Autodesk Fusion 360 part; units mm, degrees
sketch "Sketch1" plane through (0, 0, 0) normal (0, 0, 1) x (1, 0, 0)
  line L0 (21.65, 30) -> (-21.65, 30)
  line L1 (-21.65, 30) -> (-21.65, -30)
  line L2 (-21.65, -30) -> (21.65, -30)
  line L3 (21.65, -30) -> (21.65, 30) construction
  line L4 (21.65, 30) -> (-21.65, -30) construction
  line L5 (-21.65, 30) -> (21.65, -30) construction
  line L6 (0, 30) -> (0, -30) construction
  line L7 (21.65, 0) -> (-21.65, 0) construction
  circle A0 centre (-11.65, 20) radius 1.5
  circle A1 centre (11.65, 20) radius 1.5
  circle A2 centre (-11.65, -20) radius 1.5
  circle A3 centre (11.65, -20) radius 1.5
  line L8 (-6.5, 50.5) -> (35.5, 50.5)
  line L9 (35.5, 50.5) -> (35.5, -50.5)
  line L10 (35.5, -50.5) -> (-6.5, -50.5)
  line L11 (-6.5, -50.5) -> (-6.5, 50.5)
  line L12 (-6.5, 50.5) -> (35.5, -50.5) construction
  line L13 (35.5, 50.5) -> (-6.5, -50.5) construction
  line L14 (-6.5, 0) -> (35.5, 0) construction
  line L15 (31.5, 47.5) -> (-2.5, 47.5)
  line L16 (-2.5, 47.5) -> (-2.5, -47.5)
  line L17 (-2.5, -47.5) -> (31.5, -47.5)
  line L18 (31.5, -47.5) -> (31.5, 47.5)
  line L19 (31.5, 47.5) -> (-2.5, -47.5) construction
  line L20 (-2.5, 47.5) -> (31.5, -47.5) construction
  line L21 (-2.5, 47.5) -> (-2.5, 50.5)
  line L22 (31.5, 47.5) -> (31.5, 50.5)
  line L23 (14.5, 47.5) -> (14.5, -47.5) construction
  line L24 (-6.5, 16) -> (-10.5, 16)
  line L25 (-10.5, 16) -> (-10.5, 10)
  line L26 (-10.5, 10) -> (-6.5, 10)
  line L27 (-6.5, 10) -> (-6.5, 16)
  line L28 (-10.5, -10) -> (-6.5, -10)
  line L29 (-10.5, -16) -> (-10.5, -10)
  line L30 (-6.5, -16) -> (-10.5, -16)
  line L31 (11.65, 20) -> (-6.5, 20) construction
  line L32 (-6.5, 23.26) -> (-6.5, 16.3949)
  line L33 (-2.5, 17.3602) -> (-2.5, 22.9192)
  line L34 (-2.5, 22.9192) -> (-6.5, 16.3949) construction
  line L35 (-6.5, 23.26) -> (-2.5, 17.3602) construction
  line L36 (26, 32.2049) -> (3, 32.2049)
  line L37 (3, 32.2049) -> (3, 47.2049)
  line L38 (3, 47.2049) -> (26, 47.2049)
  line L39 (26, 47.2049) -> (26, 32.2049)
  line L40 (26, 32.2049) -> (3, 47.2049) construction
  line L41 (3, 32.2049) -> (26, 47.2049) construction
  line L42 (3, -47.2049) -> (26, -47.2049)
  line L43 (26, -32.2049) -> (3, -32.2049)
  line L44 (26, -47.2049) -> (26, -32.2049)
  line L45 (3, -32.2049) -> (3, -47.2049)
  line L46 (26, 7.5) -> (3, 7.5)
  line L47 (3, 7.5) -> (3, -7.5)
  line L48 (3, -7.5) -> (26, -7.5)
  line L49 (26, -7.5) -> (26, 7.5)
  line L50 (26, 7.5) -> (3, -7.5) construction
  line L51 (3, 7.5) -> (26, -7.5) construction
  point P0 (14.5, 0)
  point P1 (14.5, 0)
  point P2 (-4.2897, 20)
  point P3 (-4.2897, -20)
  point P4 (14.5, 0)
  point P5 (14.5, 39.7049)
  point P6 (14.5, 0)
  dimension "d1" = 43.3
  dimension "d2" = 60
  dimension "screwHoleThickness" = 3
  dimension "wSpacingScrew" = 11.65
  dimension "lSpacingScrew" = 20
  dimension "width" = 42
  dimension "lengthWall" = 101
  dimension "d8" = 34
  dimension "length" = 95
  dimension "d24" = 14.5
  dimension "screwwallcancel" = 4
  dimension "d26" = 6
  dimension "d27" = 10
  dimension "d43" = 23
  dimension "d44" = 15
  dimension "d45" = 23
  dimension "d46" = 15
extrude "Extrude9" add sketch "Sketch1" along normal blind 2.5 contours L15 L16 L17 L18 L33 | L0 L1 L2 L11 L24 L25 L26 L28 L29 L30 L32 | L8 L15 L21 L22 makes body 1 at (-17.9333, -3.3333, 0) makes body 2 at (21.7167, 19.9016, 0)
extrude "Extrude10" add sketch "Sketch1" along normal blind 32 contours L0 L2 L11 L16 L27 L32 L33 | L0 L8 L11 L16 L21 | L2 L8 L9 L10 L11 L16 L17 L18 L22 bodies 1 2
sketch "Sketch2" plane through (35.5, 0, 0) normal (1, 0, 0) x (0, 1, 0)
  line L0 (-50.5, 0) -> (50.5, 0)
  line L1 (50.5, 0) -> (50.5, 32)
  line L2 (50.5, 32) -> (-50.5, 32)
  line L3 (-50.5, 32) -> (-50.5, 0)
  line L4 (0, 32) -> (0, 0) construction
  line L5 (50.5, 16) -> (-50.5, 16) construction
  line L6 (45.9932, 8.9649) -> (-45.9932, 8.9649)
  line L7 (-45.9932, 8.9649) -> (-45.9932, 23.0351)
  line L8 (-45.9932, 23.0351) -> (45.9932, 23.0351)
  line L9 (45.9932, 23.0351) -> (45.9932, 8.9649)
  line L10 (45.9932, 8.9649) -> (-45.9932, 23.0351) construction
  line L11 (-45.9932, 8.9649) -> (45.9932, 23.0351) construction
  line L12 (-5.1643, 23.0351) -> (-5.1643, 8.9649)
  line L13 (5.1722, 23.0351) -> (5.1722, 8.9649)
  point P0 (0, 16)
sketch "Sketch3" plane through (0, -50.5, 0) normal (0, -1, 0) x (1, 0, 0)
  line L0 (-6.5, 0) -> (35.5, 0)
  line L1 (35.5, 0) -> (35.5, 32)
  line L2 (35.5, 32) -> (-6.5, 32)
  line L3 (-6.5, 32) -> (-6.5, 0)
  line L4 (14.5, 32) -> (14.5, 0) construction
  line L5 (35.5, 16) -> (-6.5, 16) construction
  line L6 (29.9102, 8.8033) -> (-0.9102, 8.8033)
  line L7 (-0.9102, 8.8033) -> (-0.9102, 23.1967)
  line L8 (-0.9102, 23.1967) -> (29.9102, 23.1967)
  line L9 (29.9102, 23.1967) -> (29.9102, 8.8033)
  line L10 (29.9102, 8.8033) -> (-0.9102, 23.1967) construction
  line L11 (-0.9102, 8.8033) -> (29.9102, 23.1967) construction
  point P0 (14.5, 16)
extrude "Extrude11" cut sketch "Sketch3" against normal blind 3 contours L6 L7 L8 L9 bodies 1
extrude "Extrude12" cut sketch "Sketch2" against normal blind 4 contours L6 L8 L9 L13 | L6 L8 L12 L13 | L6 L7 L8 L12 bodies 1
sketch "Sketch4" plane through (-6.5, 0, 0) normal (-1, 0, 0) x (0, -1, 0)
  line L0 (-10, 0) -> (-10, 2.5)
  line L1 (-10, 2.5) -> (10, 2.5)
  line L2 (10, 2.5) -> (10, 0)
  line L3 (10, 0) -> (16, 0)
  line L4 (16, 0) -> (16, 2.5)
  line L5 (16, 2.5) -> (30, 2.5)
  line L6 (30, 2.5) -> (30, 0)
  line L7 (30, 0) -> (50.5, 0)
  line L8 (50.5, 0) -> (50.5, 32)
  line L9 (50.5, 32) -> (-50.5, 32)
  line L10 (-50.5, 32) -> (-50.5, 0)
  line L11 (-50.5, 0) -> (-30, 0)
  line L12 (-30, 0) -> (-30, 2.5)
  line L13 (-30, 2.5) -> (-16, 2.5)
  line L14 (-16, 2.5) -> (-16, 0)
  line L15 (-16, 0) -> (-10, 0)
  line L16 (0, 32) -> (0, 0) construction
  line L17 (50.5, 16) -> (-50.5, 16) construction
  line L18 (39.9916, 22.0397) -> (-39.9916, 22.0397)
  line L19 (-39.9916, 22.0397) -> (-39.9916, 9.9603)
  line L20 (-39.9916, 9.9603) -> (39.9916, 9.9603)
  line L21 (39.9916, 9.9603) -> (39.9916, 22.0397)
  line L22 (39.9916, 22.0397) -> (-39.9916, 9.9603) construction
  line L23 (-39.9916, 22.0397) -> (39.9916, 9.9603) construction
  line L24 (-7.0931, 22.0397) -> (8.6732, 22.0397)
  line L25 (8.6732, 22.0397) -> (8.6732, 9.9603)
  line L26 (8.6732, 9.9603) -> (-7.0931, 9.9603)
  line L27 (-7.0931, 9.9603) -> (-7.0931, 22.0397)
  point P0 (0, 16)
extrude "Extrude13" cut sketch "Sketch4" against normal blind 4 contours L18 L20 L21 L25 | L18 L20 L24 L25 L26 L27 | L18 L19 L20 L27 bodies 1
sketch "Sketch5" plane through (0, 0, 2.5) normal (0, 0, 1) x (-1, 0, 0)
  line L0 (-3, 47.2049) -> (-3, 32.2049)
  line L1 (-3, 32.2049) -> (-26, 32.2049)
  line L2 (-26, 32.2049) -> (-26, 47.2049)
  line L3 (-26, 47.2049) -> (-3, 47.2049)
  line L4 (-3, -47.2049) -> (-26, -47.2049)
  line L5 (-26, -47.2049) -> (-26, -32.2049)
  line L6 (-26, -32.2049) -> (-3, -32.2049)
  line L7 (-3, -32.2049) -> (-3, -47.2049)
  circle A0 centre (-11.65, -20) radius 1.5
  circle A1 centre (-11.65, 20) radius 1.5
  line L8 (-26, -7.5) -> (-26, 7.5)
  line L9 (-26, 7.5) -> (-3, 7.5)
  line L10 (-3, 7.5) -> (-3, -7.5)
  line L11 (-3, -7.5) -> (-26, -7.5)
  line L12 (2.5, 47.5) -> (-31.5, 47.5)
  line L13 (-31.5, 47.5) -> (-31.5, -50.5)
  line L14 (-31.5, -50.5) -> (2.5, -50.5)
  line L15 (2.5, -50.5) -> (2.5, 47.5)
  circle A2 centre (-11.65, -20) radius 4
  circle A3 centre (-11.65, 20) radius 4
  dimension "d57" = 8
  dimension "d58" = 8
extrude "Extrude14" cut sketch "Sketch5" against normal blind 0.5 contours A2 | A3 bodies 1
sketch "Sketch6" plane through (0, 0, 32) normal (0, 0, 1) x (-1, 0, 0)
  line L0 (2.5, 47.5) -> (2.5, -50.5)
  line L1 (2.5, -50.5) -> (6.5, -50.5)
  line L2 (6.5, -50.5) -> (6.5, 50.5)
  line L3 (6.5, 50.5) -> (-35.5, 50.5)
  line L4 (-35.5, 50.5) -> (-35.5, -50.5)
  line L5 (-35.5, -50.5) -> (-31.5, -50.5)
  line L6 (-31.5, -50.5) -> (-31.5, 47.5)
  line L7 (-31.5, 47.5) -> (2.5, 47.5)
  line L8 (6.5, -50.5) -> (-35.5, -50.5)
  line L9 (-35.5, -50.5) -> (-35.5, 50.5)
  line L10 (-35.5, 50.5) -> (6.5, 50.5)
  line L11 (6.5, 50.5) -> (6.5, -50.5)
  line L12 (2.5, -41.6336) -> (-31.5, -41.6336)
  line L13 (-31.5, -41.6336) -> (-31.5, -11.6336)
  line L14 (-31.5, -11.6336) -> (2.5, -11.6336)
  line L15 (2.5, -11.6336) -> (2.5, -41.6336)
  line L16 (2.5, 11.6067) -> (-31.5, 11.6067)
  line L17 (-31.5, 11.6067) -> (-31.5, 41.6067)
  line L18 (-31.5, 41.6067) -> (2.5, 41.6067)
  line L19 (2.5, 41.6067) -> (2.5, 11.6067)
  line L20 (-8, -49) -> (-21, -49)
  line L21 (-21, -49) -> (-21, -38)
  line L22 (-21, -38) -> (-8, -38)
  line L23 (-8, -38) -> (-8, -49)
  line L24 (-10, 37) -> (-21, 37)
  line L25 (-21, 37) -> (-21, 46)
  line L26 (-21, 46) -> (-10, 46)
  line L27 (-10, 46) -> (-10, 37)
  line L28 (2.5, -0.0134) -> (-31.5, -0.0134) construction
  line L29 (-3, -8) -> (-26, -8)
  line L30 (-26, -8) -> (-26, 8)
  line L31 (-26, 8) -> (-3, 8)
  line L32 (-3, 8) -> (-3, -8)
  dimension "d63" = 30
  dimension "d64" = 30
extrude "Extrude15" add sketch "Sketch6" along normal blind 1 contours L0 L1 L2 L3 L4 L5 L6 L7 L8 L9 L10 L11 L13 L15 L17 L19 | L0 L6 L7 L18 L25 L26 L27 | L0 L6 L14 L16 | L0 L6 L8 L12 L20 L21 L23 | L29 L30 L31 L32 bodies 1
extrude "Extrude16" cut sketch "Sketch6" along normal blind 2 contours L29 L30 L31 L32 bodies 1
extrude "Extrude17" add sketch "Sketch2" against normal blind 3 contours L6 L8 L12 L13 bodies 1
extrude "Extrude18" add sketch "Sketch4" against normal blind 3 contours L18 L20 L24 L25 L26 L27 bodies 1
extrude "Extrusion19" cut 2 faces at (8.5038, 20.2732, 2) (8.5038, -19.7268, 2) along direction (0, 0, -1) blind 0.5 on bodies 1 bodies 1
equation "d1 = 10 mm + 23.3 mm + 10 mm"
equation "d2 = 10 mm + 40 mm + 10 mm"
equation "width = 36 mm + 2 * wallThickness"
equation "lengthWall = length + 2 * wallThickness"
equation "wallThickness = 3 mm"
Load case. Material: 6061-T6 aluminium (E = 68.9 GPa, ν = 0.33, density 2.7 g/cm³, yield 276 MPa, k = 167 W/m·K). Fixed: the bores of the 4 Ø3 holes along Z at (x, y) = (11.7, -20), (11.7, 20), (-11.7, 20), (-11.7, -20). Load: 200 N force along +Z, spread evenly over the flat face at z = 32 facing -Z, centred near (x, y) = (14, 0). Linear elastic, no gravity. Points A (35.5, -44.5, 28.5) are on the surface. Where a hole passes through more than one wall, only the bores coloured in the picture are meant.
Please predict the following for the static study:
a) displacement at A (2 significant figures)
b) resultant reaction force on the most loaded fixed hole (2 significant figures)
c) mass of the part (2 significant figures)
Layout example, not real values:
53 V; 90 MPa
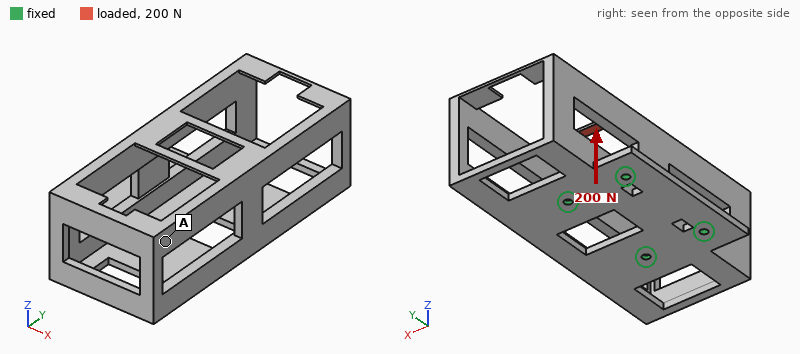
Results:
0.070 mm; 110 N; 79 g
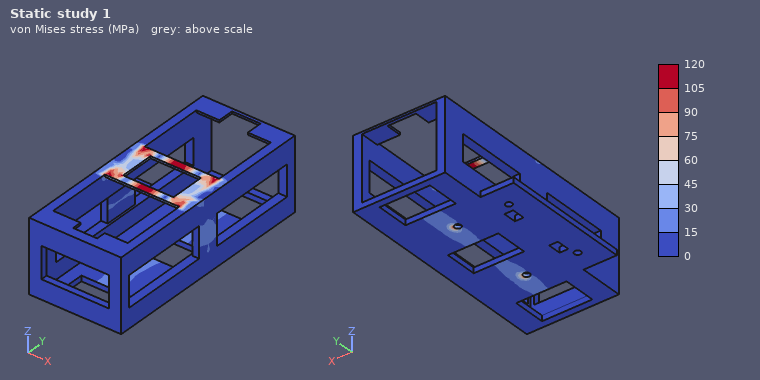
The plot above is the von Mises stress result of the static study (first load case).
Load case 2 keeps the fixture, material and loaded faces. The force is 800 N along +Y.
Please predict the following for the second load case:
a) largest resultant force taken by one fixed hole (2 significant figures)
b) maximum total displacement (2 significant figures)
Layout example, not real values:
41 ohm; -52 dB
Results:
390 N; 0.27 mm
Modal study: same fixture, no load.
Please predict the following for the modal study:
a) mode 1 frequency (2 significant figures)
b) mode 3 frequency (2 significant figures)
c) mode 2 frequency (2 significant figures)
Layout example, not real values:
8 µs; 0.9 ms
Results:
990 Hz; 1900 Hz; 1400 Hz
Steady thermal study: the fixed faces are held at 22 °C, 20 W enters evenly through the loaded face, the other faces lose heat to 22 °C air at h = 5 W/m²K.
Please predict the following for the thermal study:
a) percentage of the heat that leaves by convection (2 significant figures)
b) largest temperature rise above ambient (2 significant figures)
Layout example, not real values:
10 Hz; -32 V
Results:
7.7 %; 65 K
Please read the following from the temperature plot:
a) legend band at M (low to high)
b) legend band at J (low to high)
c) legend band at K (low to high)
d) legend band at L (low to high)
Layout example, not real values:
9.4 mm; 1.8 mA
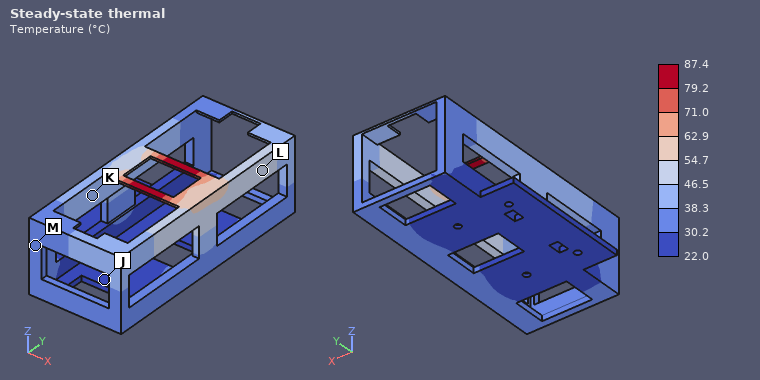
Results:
30.2 to 38.3 °C; 22.0 to 30.2 °C; 38.3 to 46.5 °C; 46.5 to 54.7 °C
